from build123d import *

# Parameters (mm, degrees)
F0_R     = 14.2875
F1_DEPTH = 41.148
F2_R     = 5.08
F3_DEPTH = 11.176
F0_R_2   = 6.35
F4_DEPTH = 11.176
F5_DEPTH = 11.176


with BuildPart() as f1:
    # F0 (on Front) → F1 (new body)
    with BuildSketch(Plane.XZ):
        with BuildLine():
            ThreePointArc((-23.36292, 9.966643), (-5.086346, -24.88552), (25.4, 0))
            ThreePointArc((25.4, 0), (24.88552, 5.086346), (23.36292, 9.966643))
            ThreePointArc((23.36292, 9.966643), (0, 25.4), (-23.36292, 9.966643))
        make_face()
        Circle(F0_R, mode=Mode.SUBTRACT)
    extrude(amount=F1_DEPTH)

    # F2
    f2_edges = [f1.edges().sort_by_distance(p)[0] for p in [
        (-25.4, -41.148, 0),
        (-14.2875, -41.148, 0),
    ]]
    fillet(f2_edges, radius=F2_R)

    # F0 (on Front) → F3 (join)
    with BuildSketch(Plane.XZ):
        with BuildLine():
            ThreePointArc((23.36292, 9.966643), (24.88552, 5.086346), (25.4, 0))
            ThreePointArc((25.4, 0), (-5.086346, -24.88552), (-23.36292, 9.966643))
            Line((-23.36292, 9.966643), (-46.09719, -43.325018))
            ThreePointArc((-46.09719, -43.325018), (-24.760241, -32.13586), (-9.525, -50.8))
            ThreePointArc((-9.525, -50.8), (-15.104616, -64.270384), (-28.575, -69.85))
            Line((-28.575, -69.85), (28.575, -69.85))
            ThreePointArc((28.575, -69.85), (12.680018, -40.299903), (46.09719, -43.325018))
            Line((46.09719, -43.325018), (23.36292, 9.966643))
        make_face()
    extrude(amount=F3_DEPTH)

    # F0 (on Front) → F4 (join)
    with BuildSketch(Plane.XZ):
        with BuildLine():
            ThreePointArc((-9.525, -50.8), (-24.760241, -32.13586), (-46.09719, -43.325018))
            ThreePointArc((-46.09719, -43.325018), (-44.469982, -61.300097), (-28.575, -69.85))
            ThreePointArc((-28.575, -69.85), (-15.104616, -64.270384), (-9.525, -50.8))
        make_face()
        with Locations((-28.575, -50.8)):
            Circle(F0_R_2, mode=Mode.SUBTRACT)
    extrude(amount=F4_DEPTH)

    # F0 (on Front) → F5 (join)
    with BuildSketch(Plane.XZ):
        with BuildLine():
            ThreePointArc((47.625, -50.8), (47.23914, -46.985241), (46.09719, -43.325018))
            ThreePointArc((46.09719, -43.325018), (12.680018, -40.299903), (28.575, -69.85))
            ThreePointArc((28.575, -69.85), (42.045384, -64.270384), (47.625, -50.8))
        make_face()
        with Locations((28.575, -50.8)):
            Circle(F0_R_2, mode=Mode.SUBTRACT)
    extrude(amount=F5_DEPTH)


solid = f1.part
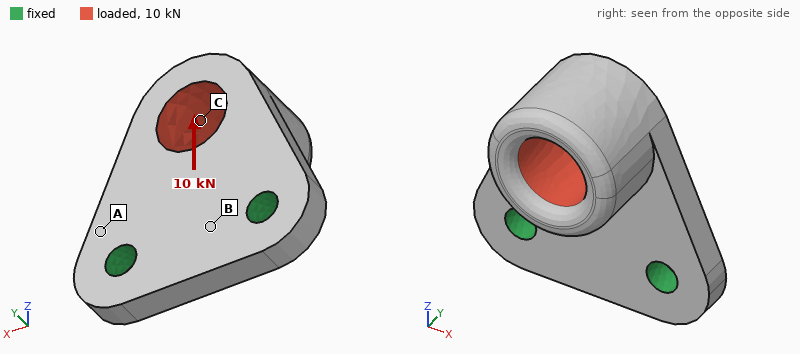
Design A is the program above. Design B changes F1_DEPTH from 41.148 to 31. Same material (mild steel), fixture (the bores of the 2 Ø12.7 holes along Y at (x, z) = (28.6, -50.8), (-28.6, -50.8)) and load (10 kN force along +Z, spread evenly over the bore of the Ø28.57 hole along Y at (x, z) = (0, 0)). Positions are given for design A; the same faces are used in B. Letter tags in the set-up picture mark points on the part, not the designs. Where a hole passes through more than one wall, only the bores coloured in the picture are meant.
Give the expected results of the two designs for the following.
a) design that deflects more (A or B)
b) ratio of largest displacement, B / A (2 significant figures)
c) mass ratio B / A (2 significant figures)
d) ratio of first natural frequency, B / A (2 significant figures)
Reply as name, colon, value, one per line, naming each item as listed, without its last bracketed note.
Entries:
design that deflects more: A
ratio of largest displacement, B / A: 0.56
mass ratio B / A: 0.86
ratio of first natural frequency, B / A: 1.2
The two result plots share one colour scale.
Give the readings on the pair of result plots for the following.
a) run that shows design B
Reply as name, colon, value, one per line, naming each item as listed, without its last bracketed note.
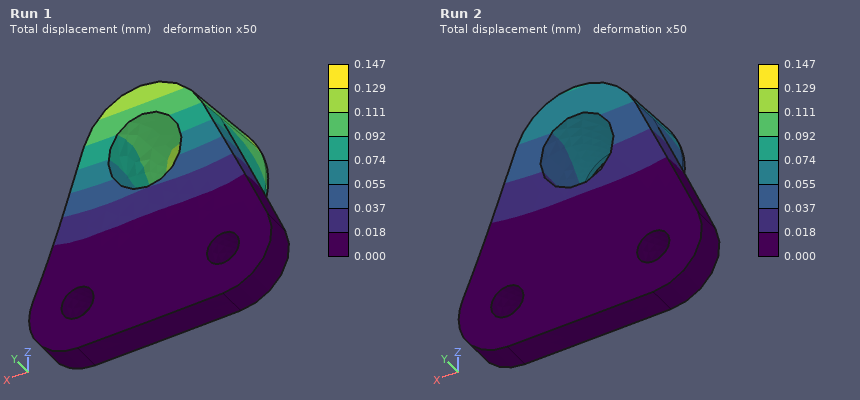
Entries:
run that shows design B: Run 2
